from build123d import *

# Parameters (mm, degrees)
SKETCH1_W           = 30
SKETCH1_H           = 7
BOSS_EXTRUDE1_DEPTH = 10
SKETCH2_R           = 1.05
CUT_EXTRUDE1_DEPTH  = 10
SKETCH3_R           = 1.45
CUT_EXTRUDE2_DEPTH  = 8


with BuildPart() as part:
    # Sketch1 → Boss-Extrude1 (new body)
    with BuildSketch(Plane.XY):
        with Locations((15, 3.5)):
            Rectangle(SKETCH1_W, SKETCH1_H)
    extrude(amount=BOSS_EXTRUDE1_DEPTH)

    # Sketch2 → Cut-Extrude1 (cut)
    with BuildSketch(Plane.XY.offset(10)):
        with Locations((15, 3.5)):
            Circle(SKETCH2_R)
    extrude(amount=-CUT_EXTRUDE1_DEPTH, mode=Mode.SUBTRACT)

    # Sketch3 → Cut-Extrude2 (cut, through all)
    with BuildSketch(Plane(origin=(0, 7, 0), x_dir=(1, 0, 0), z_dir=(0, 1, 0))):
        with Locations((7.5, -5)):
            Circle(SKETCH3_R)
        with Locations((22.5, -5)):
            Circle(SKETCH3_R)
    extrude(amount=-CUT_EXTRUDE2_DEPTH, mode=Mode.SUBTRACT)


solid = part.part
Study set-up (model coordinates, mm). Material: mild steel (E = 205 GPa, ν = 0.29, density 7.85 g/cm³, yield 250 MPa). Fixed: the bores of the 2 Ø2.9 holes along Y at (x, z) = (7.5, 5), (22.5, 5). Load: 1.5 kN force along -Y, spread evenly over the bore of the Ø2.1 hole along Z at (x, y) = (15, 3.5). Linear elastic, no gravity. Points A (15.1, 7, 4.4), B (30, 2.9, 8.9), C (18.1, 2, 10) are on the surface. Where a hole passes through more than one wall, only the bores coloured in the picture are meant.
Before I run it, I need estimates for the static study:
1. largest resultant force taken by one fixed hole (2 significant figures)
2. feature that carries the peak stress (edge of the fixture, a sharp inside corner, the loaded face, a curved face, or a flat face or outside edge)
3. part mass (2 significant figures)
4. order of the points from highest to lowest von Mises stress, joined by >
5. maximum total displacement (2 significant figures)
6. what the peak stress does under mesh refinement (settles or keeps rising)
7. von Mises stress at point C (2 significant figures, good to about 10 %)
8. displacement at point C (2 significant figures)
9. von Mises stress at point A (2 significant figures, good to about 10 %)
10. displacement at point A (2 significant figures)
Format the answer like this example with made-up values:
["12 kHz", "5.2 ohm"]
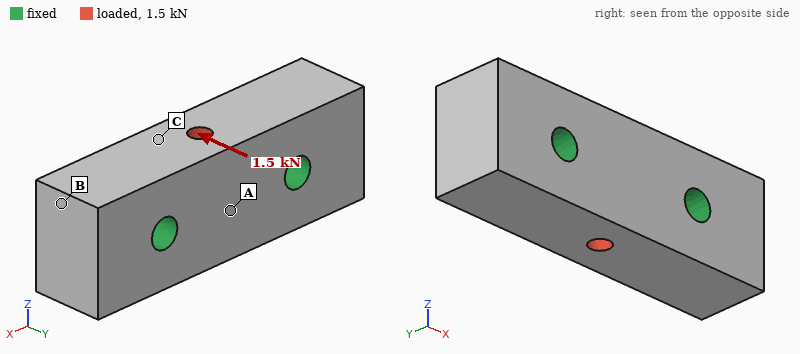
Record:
["750 N", "edge of the fixture", "15 g", "A > C > B", "1.6 µm", "keeps rising", "21 MPa", "1.0 µm", "35 MPa", "1.3 µm"]
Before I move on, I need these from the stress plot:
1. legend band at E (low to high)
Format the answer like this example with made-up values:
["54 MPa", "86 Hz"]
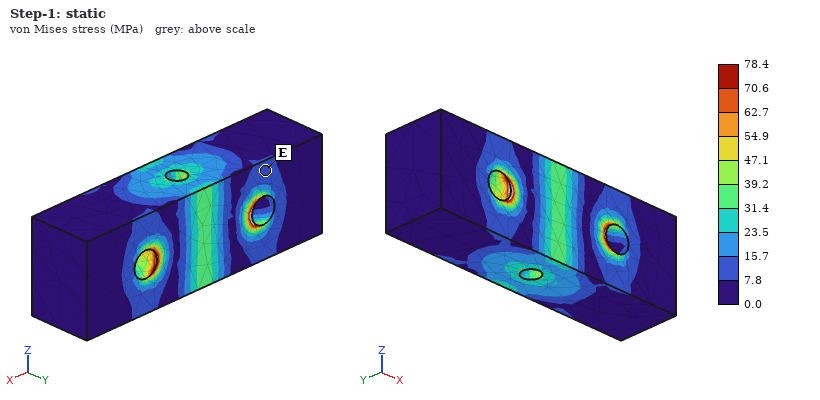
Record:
["7.8 to 15.7 MPa"]
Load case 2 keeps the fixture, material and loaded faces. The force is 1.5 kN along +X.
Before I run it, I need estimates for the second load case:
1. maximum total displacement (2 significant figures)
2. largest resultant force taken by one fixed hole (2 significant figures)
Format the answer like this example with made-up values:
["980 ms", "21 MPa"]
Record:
["0.53 µm", "750 N"]
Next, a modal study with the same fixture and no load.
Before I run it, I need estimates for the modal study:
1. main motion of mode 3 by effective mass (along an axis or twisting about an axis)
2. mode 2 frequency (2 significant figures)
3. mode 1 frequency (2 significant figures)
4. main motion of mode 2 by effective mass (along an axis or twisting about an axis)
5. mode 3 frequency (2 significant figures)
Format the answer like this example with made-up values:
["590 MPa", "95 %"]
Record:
["along Y", "63 kHz", "60 kHz", "twisting about Y", "69 kHz"]
